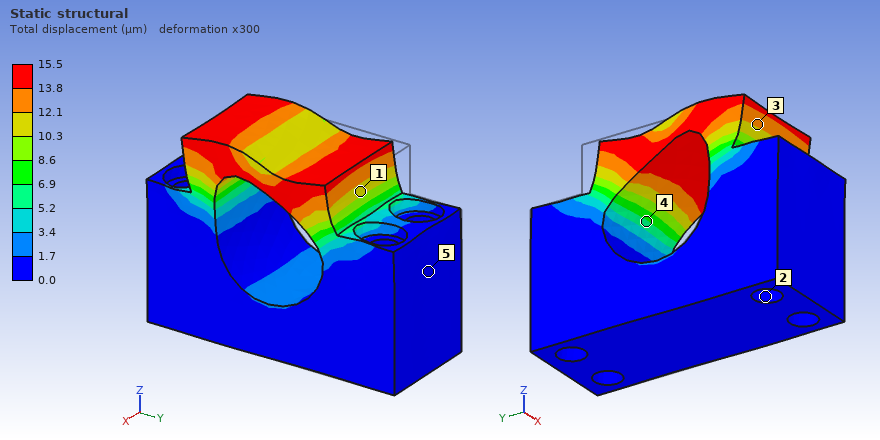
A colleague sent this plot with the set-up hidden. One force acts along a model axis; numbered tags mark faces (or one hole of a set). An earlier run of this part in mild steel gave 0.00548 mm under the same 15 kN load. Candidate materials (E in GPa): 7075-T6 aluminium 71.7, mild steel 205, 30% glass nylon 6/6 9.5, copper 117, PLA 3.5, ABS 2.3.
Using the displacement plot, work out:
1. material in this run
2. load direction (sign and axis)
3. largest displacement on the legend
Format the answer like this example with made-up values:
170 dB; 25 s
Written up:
7075-T6 aluminium; -Y; 15.5 µm
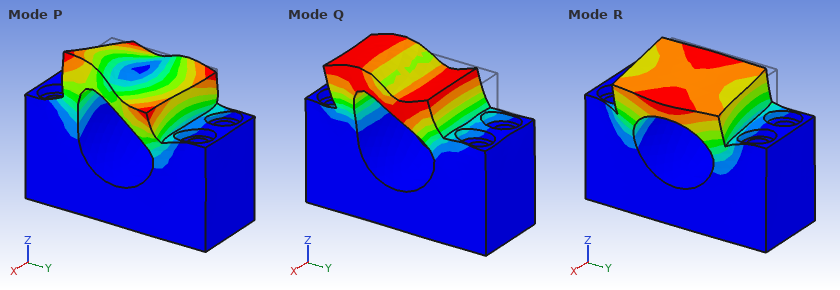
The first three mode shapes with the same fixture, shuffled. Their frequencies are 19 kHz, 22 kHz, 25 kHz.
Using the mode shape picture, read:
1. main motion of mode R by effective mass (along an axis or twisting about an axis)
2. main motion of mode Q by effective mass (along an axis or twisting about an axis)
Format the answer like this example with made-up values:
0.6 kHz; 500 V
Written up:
along X; along Y
